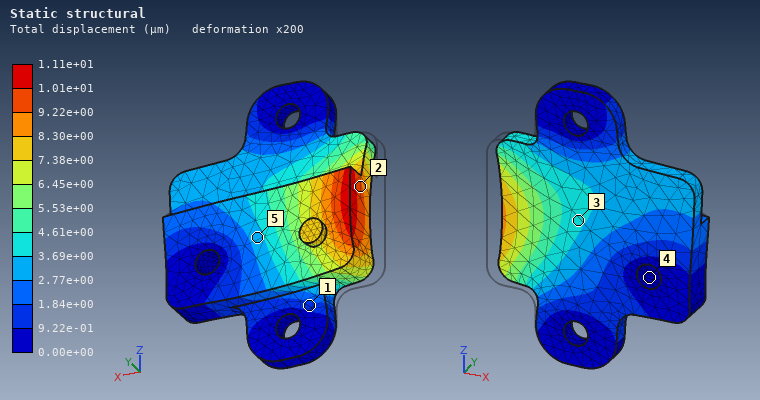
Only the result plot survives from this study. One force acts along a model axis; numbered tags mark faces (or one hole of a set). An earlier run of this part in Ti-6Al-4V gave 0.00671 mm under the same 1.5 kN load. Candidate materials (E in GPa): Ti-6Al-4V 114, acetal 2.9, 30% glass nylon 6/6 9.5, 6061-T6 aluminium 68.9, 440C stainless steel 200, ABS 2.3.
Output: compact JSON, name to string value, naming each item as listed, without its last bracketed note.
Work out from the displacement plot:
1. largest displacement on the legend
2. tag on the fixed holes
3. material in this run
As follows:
{"largest displacement on the legend": "1.11e+01 µm", "tag on the fixed holes": "4", "material in this run": "6061-T6 aluminium"}
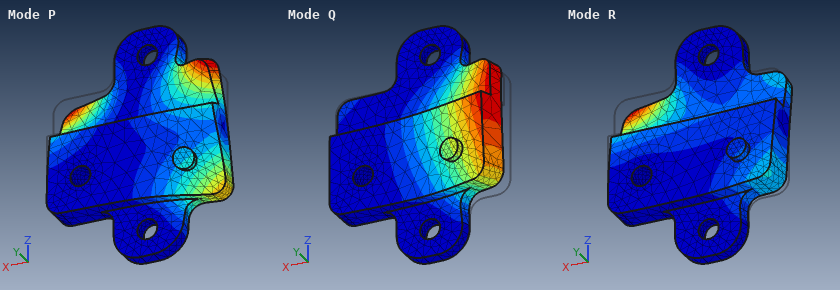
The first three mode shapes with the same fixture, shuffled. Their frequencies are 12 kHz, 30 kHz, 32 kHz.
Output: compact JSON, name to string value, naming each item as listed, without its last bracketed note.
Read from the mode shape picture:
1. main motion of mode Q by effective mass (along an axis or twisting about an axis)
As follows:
{"main motion of mode Q by effective mass": "along Y"}
